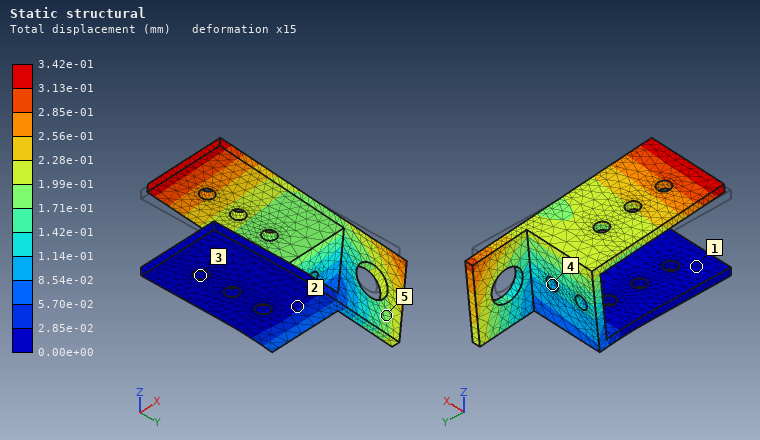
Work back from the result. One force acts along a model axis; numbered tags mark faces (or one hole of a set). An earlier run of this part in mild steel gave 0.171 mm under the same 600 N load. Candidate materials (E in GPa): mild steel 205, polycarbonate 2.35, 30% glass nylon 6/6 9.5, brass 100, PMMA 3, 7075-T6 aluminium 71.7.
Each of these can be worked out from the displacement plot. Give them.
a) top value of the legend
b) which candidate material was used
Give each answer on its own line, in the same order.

3.42e-01 mm
brass
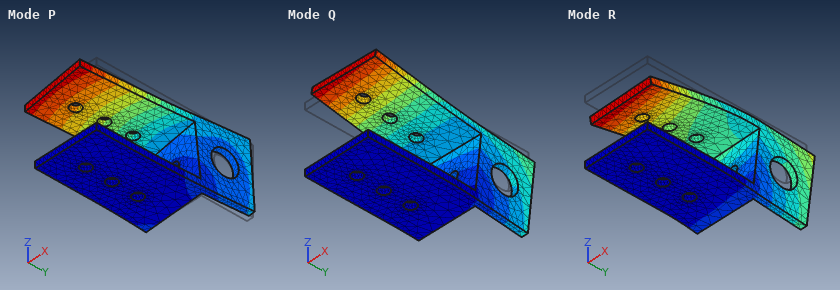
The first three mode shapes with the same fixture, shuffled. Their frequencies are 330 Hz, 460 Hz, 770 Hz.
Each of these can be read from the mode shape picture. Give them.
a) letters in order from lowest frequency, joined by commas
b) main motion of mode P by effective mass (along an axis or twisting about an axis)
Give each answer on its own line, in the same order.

Q, P, R
along X
